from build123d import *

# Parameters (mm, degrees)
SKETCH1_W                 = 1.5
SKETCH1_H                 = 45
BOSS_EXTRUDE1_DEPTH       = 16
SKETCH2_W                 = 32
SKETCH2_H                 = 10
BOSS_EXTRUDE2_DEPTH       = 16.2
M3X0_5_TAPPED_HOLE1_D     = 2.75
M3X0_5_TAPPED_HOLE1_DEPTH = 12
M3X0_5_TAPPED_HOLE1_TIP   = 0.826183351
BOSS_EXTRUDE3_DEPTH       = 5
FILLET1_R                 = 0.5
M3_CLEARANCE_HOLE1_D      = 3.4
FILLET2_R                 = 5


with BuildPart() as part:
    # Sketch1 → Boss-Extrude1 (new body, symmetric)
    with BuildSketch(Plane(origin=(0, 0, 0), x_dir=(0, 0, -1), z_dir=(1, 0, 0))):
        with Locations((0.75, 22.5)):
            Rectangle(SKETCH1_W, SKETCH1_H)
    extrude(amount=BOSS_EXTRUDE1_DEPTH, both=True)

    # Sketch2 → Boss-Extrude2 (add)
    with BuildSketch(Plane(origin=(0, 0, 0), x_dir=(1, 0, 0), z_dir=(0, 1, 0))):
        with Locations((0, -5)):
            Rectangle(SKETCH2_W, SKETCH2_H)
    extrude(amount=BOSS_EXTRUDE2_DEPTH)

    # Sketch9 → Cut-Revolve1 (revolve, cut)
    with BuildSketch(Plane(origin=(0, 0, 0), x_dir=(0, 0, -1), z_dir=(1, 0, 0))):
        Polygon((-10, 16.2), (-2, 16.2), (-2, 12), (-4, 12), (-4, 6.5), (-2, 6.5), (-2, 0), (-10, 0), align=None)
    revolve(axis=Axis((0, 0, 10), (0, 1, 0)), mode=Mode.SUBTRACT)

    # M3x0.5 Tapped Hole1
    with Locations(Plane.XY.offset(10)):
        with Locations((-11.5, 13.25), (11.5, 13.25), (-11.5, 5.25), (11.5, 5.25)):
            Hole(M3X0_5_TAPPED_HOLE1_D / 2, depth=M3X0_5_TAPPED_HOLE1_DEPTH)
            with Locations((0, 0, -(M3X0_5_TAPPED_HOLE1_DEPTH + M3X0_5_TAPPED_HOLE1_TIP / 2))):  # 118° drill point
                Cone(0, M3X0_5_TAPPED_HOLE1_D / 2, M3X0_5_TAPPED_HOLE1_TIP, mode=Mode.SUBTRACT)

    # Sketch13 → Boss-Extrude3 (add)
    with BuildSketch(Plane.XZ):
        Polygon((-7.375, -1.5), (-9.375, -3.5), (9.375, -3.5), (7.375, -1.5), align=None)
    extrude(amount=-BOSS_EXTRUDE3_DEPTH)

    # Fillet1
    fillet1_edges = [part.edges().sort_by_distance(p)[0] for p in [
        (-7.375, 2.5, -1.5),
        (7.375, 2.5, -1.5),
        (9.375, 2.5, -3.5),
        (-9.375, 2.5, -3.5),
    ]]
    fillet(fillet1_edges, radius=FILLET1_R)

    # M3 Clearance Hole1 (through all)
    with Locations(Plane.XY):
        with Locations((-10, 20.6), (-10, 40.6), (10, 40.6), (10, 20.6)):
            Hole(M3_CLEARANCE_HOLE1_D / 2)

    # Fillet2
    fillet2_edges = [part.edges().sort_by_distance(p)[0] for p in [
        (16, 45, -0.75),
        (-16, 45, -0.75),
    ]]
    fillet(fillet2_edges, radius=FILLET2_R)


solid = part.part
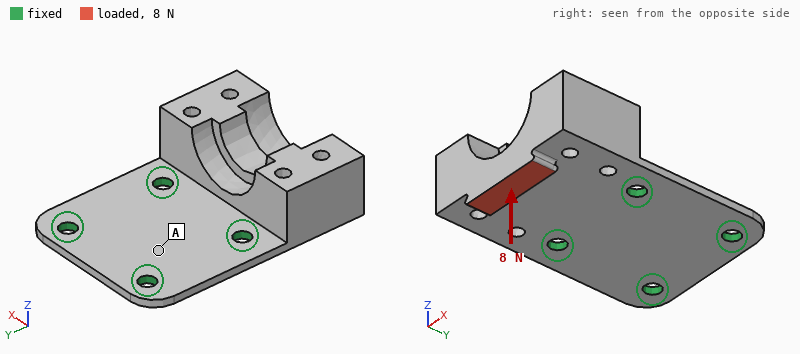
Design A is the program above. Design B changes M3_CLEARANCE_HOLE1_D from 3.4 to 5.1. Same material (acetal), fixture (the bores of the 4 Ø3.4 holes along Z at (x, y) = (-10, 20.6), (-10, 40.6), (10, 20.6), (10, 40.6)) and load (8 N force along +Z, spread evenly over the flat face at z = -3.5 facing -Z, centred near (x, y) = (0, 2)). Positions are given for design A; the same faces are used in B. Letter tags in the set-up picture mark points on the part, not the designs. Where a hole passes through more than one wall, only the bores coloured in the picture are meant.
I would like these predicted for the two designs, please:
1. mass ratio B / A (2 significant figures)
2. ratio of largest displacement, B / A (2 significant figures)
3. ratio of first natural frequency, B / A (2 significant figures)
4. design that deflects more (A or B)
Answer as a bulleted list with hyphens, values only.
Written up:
- 0.99
- 0.72
- 1.2
- A
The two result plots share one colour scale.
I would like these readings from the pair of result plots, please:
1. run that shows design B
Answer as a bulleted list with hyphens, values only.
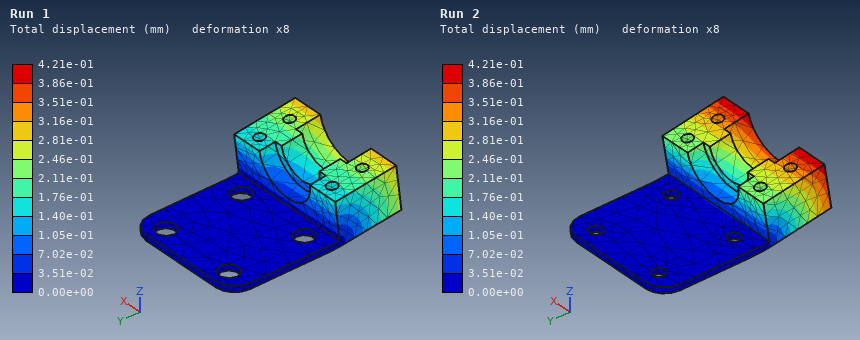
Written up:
- Run 1
